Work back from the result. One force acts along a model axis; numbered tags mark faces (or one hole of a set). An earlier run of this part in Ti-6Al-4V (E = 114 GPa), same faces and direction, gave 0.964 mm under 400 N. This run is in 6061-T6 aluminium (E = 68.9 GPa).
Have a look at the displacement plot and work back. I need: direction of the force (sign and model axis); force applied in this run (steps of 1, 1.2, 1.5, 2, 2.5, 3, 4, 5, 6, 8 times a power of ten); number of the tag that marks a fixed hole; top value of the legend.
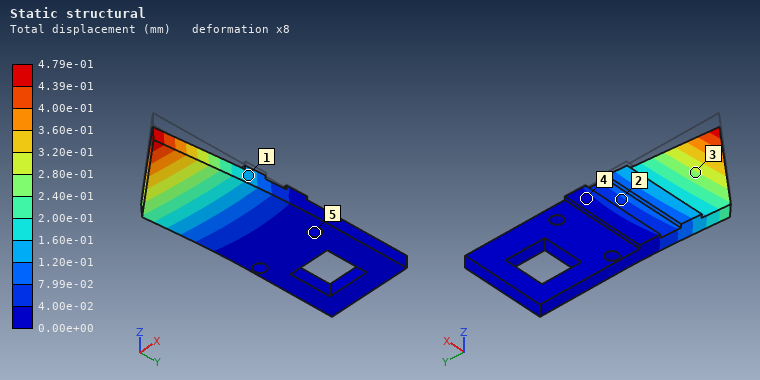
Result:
-Z
120 N
5
4.79e-01 mm
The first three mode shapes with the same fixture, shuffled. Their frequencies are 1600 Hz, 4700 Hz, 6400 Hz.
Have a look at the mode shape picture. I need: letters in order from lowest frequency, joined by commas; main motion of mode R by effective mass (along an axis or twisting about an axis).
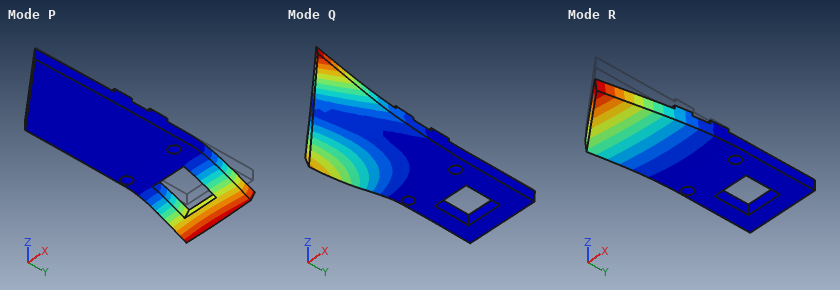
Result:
R, P, Q
along Z
